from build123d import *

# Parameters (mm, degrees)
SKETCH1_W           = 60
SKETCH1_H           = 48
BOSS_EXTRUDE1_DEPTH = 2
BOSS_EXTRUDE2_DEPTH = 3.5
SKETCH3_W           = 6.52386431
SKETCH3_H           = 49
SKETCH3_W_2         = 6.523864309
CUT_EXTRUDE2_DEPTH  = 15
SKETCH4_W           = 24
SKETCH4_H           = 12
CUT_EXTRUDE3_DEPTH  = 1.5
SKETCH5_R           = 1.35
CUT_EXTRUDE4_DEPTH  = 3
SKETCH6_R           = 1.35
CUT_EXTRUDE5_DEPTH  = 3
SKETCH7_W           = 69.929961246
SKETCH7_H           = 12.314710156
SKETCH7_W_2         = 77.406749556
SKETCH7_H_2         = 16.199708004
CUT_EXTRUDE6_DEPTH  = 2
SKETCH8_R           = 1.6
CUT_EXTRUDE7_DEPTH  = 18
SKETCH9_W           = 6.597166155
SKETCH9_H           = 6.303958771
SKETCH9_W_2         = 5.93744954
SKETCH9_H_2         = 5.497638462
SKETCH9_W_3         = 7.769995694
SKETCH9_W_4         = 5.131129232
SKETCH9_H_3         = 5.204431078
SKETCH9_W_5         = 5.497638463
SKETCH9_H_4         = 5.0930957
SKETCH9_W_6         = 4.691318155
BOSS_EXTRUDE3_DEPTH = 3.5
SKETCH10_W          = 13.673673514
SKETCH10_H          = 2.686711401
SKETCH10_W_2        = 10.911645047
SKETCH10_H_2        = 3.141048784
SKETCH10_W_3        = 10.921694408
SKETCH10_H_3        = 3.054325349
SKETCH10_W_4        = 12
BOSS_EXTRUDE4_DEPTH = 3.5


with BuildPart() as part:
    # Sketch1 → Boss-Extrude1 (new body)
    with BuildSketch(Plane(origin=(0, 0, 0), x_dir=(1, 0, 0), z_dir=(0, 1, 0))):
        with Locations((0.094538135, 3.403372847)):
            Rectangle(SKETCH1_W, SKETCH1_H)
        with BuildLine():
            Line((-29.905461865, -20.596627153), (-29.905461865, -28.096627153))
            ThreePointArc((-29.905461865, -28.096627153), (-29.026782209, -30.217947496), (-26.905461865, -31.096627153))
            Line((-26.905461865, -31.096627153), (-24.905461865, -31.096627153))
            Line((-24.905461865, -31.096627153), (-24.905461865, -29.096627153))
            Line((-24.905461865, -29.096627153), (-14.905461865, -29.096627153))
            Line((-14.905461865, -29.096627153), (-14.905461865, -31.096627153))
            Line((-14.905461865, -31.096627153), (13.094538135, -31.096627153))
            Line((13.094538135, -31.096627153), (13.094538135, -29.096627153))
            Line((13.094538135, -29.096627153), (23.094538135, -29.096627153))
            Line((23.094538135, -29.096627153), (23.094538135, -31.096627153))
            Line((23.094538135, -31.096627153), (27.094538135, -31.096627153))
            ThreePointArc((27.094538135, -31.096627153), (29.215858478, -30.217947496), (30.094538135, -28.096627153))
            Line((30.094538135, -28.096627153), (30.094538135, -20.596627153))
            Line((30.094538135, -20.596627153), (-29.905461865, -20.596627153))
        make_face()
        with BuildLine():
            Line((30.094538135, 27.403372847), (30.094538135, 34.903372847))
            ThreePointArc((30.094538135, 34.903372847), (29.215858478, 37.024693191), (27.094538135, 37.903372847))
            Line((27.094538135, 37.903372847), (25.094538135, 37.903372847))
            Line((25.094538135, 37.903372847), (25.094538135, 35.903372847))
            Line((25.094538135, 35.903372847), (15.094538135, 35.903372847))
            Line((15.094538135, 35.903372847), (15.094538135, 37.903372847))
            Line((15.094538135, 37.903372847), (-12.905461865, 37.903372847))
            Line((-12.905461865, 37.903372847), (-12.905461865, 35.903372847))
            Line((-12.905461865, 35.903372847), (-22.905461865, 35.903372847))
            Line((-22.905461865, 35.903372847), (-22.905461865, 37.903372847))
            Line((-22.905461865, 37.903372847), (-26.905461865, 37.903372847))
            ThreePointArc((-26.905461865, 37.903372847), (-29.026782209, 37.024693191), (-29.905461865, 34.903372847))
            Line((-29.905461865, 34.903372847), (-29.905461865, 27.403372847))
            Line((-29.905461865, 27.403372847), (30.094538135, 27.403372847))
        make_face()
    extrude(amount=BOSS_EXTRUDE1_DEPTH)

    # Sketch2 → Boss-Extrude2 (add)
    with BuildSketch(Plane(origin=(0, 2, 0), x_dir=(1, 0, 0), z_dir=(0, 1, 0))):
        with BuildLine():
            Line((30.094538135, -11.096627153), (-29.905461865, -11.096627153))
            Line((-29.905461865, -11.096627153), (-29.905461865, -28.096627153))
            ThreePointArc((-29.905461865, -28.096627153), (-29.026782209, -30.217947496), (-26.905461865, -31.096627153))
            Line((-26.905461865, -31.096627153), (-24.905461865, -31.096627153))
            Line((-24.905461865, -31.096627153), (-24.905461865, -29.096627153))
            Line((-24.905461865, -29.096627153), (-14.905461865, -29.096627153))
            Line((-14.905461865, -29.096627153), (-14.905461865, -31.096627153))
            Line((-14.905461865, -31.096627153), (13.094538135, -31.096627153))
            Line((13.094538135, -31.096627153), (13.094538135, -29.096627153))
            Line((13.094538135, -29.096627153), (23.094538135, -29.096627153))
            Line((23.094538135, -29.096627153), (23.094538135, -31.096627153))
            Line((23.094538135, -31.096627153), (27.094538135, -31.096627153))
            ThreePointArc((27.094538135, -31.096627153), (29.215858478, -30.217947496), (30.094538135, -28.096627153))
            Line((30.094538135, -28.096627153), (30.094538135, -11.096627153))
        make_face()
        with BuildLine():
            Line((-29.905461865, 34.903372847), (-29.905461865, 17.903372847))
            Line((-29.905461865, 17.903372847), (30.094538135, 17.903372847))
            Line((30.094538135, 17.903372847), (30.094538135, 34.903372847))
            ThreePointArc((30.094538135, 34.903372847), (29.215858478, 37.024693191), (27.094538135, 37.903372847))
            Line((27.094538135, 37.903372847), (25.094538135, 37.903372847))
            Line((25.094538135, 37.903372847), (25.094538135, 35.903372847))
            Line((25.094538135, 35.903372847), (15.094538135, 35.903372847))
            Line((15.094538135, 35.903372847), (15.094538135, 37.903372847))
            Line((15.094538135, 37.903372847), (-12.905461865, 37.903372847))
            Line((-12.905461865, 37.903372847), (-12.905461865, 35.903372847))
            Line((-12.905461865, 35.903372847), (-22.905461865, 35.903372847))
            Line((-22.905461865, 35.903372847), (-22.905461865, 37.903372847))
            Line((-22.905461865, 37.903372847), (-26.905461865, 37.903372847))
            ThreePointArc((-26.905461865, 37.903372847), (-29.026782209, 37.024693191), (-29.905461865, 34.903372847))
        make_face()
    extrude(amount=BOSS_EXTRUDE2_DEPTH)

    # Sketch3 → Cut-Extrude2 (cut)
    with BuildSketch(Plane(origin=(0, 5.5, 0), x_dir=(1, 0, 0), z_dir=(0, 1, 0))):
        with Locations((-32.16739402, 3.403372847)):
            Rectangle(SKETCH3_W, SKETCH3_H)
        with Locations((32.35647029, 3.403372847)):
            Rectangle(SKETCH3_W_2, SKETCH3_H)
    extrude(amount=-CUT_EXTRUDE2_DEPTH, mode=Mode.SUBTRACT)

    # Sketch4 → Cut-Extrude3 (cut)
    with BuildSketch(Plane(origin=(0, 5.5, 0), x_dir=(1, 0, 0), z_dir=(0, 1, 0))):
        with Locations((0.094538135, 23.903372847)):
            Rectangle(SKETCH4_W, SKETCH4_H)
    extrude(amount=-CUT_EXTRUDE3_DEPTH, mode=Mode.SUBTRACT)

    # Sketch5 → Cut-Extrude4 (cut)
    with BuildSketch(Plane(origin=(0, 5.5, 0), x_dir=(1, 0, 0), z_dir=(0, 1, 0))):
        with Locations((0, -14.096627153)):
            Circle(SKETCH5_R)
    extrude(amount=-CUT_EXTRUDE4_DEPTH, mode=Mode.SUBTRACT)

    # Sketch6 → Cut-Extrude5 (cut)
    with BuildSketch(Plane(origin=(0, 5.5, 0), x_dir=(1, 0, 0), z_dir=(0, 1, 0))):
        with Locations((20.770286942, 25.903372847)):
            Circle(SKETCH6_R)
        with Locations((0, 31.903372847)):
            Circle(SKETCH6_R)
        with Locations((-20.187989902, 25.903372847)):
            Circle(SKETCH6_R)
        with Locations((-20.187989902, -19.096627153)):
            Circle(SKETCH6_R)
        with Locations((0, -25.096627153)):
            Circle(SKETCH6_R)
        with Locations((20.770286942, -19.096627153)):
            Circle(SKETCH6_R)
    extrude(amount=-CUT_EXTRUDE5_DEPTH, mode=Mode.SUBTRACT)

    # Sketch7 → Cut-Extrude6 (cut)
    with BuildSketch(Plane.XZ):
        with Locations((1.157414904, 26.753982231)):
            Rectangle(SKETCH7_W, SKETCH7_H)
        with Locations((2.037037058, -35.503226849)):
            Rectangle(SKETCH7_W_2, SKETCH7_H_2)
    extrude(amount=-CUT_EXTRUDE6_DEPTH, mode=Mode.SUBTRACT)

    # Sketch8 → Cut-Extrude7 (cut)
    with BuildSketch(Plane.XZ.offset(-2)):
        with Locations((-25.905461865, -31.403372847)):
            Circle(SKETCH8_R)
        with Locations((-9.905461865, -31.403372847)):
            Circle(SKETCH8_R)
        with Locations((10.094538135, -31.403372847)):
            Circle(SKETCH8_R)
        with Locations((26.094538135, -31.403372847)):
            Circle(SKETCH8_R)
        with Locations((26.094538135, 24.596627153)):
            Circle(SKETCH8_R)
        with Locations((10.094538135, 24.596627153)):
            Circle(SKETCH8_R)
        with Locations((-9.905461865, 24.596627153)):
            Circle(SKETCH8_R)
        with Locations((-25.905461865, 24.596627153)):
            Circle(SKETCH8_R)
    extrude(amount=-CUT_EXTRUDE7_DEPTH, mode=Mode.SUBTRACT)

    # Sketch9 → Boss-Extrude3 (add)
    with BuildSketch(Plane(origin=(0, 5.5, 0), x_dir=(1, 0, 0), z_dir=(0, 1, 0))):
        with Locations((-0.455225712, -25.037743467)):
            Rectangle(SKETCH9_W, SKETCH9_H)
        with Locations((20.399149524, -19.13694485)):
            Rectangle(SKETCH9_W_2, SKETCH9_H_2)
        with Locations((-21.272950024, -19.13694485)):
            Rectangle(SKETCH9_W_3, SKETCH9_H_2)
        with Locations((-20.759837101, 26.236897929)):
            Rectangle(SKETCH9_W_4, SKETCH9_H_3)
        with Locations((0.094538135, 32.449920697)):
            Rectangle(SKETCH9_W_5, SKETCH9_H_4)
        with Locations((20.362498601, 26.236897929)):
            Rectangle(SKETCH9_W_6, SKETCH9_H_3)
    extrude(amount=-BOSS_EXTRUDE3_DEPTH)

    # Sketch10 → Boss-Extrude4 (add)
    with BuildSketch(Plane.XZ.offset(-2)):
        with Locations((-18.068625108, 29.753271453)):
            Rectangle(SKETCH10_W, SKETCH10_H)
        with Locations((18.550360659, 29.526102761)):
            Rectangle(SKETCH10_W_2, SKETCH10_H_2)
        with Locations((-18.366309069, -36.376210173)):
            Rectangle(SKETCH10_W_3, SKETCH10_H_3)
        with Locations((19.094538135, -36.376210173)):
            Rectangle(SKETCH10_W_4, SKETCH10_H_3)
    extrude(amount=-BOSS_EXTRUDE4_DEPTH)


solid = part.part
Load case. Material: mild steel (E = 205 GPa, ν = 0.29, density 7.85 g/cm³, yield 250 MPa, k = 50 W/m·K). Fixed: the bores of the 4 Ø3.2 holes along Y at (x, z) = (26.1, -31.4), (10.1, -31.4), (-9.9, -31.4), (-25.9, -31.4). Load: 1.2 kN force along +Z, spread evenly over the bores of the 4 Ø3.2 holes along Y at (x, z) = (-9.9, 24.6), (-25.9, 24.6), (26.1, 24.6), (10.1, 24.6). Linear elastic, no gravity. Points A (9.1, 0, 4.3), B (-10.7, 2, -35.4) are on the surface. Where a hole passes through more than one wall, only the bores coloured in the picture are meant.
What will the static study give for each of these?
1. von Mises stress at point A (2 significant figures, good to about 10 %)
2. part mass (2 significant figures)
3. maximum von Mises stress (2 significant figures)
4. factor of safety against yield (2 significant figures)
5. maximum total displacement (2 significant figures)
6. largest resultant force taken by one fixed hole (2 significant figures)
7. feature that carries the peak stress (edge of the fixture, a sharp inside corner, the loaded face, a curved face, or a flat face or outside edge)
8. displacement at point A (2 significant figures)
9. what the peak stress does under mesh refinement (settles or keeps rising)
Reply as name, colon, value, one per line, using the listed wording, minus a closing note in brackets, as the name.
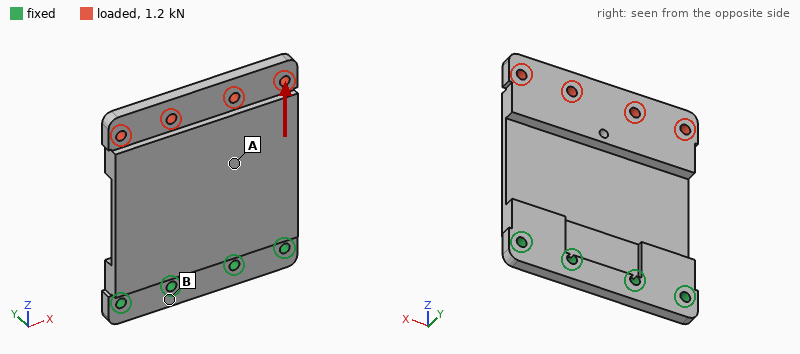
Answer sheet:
von Mises stress at point A: 67 MPa
part mass: 100 g
maximum von Mises stress: 97 MPa
factor of safety against yield: 2.6
maximum total displacement: 0.43 mm
largest resultant force taken by one fixed hole: 330 N
feature that carries the peak stress: a flat face or outside edge
displacement at point A: 0.11 mm
what the peak stress does under mesh refinement: settles
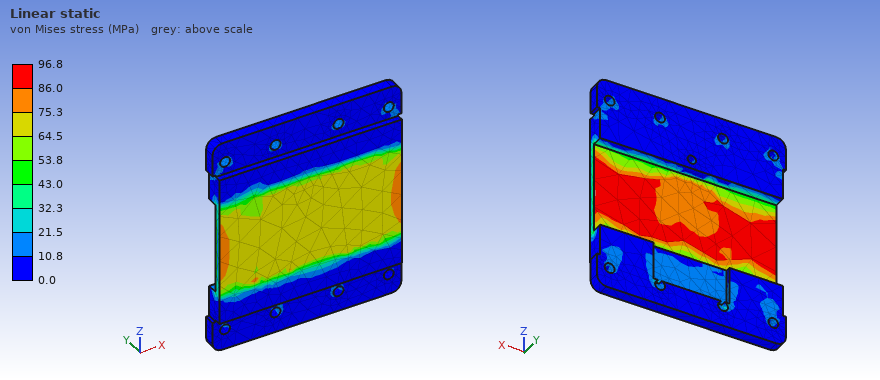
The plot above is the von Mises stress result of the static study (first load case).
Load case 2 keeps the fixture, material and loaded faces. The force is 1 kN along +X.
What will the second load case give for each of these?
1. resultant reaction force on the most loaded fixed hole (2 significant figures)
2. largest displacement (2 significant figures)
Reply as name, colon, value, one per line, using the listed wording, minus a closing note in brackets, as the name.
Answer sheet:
resultant reaction force on the most loaded fixed hole: 1.0 kN
largest displacement: 0.11 mm
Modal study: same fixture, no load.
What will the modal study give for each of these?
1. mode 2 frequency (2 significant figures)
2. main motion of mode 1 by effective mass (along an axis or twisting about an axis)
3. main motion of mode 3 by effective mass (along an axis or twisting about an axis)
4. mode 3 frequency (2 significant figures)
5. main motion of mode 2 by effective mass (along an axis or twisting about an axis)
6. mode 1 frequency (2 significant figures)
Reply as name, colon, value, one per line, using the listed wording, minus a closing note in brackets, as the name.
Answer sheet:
mode 2 frequency: 1300 Hz
main motion of mode 1 by effective mass: along Y
main motion of mode 3 by effective mass: along Y
mode 3 frequency: 3100 Hz
main motion of mode 2 by effective mass: twisting about Z
mode 1 frequency: 450 Hz
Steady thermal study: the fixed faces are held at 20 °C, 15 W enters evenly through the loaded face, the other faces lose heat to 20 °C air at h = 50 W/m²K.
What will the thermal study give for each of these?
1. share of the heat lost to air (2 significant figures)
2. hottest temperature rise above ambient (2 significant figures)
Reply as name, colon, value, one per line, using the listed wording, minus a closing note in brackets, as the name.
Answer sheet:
share of the heat lost to air: 71 %
hottest temperature rise above ambient: 56 K
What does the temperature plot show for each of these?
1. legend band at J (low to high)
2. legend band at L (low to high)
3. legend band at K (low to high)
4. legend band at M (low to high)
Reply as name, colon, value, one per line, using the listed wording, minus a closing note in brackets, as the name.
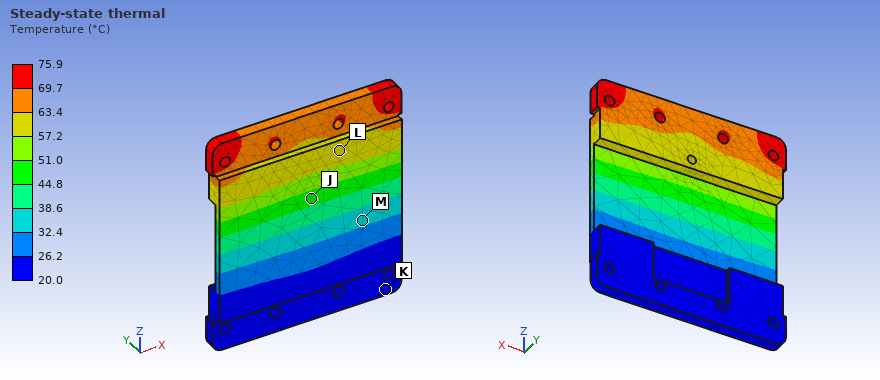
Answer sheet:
legend band at J: 44.8 to 51.0 °C
legend band at L: 57.2 to 63.4 °C
legend band at K: 20.0 to 26.2 °C
legend band at M: 32.4 to 38.6 °C
